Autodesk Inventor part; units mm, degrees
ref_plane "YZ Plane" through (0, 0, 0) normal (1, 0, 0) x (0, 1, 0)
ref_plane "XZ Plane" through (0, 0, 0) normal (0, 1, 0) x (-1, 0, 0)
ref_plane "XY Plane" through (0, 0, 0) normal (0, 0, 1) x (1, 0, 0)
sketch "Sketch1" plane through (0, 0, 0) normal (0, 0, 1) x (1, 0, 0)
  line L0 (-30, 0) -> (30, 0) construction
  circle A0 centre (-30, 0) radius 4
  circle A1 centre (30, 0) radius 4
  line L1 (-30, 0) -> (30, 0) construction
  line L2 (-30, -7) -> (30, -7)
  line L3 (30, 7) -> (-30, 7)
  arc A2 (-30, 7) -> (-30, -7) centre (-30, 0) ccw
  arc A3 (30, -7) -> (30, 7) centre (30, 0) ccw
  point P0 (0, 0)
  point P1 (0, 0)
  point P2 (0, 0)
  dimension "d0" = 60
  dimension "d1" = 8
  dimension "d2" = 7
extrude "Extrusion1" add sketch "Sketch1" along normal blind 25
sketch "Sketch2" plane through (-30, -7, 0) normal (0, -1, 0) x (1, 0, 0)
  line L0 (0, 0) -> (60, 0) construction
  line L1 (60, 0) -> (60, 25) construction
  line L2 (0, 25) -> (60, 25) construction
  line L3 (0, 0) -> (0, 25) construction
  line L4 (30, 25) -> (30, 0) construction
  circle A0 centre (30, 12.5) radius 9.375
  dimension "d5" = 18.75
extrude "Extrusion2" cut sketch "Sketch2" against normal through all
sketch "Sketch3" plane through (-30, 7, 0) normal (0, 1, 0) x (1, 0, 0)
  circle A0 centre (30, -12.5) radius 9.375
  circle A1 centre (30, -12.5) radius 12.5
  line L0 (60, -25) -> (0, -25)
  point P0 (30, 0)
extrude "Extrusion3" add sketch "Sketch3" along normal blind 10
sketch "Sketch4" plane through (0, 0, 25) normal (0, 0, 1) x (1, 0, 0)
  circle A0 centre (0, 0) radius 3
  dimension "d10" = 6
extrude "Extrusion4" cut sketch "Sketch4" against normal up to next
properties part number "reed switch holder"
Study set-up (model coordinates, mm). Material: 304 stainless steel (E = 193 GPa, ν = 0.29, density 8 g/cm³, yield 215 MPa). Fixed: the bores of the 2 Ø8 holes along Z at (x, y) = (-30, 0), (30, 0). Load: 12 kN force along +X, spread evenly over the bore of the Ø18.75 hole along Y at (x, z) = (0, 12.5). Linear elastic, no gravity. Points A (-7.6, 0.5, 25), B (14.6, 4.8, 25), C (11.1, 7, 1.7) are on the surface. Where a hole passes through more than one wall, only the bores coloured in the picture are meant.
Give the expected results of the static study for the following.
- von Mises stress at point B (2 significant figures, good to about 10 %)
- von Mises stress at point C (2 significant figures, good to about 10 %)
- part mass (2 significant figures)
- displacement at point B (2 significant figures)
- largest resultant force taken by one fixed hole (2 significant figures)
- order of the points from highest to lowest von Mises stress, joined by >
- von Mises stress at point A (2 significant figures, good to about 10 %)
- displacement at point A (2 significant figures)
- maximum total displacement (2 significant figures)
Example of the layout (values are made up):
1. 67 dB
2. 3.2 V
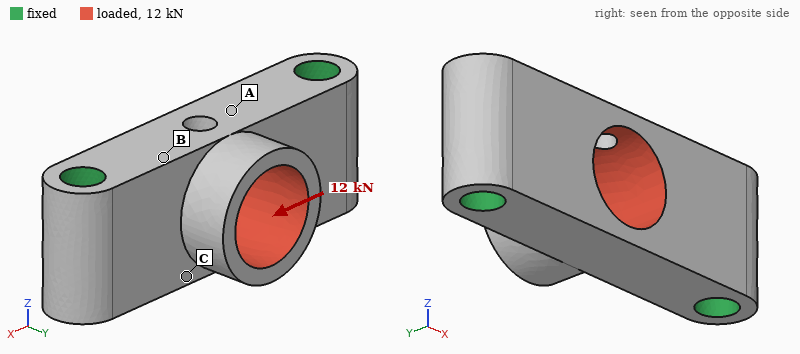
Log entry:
1. 25 MPa
2. 39 MPa
3. 160 g
4. 1.6 µm
5. 6.2 kN
6. C > B > A
7. 8.6 MPa
8. 1.9 µm
9. 9.4 µm
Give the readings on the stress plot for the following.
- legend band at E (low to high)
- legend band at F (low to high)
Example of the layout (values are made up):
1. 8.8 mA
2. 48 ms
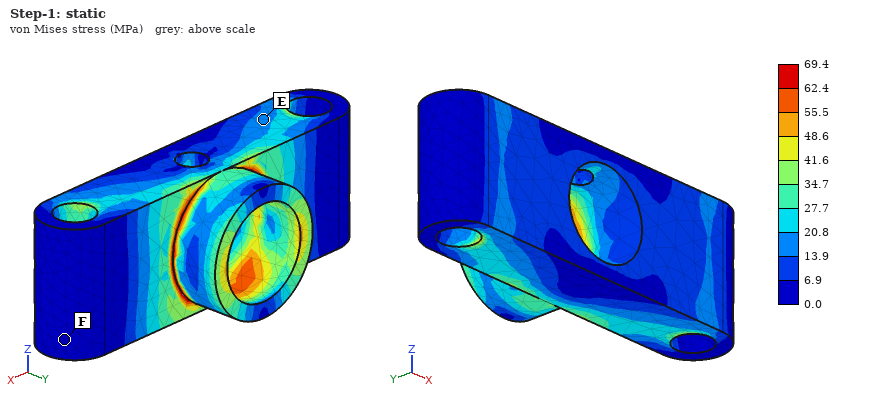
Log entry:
1. 13.9 to 20.8 MPa
2. 0.0 to 6.9 MPa
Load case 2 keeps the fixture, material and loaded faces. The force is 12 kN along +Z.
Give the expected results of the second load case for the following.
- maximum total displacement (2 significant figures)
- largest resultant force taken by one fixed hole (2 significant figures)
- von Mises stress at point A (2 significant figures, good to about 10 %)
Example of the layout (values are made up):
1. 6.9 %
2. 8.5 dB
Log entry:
1. 24 µm
2. 6.0 kN
3. 28 MPa
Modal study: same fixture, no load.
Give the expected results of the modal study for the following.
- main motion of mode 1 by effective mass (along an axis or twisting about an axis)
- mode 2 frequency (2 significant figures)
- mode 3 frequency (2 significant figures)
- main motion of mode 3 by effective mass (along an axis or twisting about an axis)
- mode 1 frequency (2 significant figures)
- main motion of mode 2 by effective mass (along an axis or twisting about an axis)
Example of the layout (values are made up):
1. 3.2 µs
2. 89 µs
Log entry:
1. along Y
2. 18 kHz
3. 26 kHz
4. along Z
5. 16 kHz
6. along Z
